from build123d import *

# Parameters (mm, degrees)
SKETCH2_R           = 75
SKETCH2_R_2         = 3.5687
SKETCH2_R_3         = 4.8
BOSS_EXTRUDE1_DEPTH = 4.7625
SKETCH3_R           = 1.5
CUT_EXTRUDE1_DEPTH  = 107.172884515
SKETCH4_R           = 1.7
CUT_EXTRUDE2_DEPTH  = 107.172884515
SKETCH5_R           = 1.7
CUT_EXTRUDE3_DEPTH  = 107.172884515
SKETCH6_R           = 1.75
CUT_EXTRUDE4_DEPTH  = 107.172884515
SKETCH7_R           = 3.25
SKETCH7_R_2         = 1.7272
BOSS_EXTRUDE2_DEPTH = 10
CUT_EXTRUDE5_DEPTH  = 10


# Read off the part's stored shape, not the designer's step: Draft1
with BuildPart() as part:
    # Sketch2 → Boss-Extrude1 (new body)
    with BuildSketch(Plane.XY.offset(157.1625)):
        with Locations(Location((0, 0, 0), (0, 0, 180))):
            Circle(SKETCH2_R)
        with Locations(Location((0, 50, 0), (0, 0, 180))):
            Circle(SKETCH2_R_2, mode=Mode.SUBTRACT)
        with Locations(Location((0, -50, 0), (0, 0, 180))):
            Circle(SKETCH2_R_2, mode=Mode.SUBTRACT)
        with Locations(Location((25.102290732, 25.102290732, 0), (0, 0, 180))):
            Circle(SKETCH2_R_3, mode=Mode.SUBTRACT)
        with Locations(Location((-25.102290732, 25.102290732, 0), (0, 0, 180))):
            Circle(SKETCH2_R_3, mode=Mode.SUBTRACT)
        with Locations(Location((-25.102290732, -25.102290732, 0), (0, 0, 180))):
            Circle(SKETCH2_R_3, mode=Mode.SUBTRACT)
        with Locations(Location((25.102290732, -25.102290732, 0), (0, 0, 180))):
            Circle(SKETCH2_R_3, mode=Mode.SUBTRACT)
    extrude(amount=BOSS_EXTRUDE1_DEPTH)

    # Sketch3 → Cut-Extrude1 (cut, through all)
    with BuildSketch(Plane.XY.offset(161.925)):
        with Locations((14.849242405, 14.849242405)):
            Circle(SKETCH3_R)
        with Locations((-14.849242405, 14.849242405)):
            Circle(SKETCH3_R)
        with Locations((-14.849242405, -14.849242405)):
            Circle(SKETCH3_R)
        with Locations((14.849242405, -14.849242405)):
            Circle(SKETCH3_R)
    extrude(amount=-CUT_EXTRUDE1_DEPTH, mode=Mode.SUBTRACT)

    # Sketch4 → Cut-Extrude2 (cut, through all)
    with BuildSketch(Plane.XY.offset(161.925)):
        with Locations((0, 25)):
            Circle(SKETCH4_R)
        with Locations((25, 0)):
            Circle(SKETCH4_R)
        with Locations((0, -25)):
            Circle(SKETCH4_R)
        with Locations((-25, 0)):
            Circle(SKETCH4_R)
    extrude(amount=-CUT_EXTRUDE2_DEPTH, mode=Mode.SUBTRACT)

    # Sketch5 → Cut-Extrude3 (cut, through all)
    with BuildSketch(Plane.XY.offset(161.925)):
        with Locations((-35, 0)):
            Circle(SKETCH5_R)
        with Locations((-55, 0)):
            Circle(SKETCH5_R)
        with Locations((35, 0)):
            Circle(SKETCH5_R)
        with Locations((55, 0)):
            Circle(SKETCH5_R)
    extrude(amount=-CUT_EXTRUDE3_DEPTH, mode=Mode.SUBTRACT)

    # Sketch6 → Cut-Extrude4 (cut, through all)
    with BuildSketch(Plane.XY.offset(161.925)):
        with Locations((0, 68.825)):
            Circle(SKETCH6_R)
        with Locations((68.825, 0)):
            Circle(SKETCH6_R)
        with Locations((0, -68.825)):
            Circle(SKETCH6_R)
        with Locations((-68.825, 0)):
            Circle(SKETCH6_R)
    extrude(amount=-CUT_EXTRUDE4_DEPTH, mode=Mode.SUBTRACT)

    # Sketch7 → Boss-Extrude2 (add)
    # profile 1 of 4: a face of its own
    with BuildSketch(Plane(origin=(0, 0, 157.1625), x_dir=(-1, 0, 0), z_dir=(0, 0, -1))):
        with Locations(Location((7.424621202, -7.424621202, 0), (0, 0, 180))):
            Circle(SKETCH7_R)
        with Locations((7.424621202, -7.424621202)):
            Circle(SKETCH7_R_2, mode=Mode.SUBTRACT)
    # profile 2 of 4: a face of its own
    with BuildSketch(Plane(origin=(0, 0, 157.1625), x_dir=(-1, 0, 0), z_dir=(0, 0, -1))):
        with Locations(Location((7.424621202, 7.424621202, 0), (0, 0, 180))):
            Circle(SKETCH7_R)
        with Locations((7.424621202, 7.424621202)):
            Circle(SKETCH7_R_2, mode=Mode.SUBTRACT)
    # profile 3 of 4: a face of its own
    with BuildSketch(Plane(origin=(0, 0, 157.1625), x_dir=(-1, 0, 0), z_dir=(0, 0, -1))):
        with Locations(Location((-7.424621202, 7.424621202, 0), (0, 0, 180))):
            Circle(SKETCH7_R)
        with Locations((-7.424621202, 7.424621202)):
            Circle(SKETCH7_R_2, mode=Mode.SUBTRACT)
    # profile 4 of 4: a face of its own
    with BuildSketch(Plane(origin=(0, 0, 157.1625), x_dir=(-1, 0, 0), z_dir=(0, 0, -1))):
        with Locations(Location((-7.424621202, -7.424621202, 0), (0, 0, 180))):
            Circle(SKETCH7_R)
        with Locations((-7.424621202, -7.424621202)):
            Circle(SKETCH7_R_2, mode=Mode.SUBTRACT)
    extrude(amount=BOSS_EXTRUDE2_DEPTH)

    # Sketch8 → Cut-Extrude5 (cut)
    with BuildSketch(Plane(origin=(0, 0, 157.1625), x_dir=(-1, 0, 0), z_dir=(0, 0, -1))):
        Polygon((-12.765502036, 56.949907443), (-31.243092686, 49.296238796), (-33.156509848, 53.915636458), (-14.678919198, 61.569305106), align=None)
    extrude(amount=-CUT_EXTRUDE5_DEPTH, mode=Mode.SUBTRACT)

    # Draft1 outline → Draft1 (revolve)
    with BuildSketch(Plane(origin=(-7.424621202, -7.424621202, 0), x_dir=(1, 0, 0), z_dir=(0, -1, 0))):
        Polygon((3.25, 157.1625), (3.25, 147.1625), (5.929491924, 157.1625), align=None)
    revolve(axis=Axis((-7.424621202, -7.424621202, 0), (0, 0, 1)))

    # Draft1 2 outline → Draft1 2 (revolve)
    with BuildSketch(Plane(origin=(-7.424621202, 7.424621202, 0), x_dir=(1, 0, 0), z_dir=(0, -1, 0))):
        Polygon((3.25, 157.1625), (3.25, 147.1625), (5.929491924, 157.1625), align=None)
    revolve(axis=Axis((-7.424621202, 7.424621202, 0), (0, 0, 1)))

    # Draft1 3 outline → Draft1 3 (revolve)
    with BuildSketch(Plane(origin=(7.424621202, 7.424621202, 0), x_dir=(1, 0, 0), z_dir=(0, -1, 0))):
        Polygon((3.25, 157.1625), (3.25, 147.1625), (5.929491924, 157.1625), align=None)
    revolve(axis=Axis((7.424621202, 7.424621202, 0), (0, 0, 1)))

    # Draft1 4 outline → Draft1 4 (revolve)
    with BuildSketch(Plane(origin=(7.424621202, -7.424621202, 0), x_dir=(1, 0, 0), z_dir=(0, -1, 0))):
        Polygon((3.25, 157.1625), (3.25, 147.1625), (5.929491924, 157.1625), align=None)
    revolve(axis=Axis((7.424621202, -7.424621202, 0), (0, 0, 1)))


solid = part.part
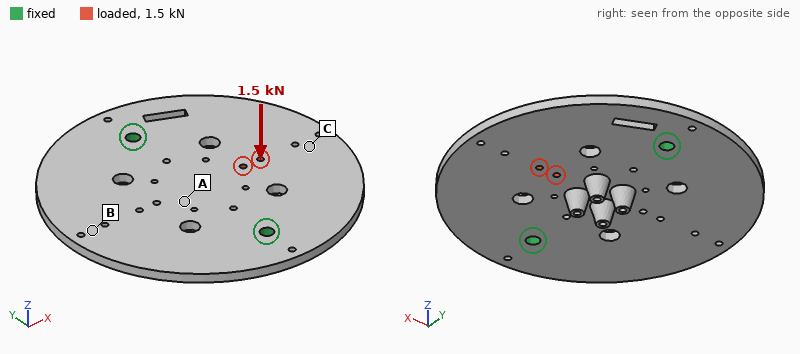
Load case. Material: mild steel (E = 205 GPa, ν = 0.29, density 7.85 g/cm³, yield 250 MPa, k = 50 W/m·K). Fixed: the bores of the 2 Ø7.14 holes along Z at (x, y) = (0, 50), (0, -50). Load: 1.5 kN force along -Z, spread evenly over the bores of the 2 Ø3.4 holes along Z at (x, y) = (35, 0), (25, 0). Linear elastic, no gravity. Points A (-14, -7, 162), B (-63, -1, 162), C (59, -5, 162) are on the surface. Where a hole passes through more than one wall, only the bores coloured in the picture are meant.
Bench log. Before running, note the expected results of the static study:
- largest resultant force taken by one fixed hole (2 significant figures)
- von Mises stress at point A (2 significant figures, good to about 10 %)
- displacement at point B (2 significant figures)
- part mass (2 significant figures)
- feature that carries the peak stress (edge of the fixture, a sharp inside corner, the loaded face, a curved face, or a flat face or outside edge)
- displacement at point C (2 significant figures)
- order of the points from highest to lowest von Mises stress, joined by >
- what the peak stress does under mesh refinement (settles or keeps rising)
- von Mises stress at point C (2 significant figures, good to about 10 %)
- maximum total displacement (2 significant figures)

770 N
33 MPa
0.082 mm
660 g
edge of the fixture
0.29 mm
C > A > B
keeps rising
49 MPa
0.37 mm
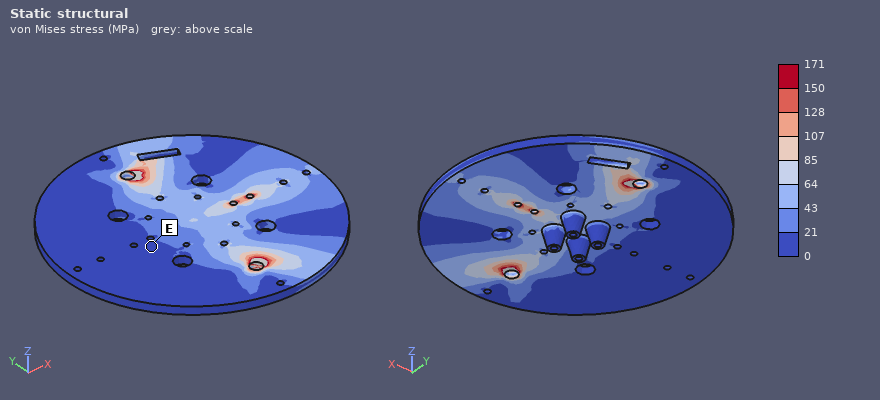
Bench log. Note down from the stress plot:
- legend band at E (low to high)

0 to 21 MPa
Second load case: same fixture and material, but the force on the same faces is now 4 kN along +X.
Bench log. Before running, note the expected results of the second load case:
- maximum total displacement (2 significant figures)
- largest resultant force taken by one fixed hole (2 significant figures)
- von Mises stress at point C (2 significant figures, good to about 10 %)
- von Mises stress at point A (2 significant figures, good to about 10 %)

6.0 µm
2.0 kN
9.2 MPa
6.5 MPa
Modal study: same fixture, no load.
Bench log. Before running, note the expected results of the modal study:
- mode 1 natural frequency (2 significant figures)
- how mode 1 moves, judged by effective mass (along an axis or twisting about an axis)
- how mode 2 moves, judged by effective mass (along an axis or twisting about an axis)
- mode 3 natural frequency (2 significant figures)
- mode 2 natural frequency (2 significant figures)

670 Hz
twisting about Y
along Z
1700 Hz
880 Hz
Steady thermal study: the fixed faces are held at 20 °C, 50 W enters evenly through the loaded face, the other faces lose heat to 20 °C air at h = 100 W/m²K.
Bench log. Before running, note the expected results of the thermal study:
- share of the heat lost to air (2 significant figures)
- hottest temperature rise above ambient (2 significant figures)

84 %
85 K
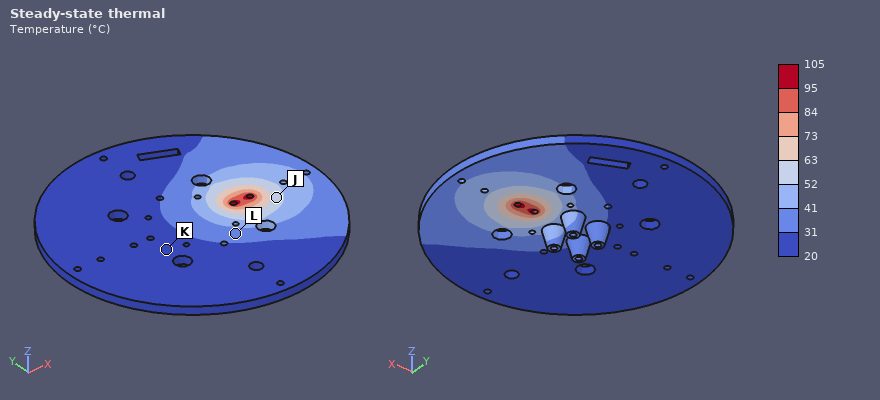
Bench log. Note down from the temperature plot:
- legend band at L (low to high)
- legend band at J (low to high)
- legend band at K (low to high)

31 to 41 °C
52 to 63 °C
20 to 31 °C
